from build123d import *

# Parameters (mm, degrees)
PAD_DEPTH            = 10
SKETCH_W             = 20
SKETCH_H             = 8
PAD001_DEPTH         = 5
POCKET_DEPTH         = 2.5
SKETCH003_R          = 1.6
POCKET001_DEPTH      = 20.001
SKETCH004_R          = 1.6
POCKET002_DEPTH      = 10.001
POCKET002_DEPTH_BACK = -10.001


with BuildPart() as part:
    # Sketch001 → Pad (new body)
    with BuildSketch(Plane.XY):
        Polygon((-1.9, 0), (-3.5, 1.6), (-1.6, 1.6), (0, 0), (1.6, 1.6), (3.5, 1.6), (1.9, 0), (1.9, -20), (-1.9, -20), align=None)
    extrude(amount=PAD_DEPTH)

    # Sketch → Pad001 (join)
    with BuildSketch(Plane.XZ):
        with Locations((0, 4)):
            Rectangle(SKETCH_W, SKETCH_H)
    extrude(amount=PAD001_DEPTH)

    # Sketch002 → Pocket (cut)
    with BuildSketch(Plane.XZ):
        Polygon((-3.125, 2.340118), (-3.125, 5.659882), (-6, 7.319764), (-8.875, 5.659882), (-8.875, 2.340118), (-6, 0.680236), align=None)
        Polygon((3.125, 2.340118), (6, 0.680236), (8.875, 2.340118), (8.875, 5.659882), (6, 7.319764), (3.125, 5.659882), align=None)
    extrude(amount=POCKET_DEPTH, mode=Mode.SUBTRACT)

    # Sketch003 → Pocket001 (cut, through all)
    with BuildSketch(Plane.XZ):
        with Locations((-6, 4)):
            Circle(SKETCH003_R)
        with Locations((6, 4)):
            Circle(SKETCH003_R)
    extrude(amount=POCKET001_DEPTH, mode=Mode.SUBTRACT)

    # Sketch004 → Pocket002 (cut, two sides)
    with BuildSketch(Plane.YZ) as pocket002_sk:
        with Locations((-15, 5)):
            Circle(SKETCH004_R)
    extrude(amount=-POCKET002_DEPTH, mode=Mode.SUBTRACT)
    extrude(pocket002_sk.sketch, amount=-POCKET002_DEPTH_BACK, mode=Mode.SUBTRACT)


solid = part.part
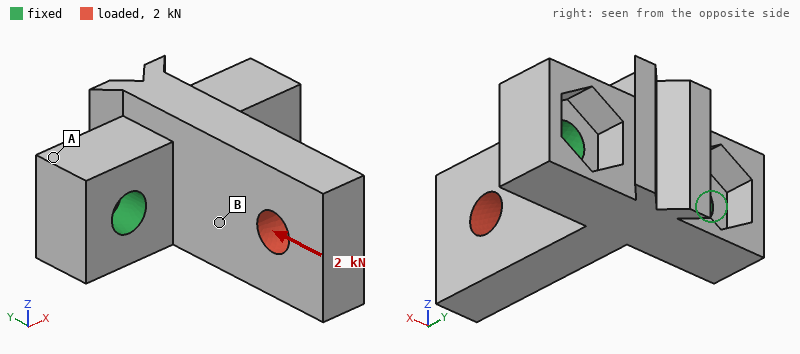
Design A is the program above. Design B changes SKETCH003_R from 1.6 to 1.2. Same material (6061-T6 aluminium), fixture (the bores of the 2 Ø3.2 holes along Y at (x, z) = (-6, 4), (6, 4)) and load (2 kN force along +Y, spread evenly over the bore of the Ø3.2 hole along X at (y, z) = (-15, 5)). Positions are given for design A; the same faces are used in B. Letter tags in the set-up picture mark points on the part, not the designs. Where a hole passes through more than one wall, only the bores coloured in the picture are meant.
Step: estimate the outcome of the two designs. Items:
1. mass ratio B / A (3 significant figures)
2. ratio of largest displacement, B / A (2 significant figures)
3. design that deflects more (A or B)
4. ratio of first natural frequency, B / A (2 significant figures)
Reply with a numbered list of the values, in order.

1. 1.01
2. 1.2
3. B
4. 0.99
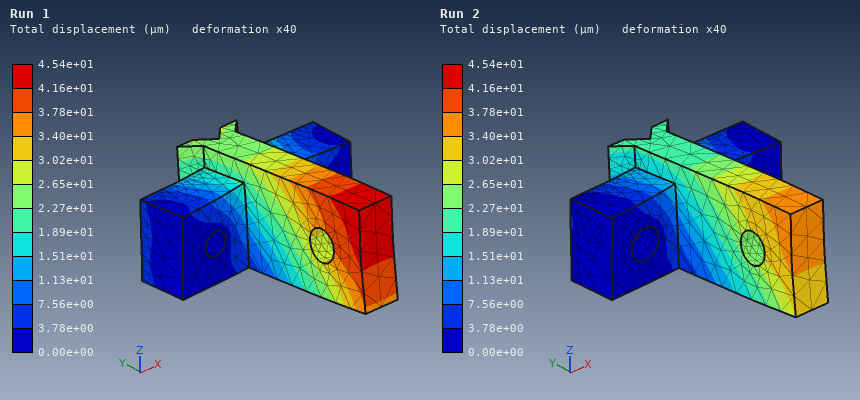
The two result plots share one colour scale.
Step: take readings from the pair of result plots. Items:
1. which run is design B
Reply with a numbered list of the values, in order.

1. Run 1
